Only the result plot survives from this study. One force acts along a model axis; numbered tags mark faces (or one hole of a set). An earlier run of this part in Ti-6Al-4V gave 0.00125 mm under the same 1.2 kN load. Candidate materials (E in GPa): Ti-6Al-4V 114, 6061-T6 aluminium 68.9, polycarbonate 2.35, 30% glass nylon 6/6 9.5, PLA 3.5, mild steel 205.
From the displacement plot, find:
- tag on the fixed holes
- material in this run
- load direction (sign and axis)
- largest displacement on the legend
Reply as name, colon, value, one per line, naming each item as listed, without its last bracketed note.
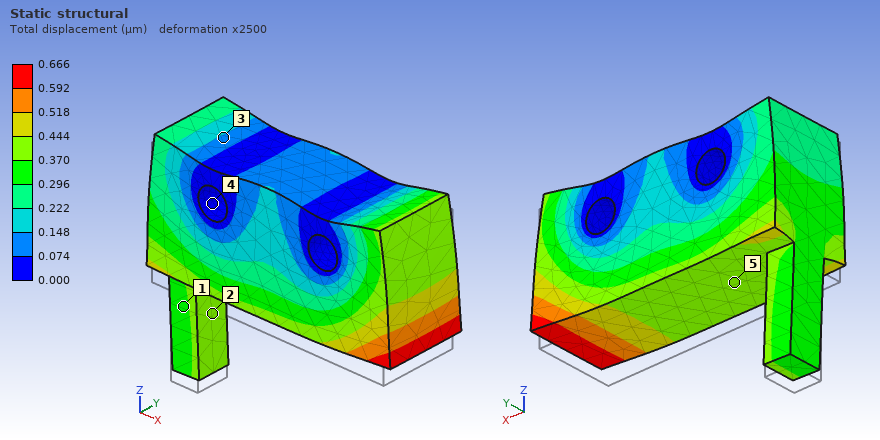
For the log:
tag on the fixed holes: 4
material in this run: mild steel
load direction: +Z
largest displacement on the legend: 0.666 µm
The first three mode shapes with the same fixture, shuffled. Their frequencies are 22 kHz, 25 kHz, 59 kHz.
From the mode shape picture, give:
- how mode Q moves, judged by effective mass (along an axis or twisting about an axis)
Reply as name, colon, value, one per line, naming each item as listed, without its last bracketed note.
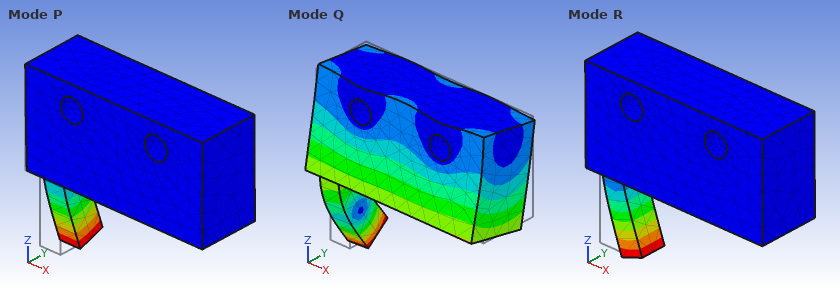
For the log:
how mode Q moves, judged by effective mass: along Y
